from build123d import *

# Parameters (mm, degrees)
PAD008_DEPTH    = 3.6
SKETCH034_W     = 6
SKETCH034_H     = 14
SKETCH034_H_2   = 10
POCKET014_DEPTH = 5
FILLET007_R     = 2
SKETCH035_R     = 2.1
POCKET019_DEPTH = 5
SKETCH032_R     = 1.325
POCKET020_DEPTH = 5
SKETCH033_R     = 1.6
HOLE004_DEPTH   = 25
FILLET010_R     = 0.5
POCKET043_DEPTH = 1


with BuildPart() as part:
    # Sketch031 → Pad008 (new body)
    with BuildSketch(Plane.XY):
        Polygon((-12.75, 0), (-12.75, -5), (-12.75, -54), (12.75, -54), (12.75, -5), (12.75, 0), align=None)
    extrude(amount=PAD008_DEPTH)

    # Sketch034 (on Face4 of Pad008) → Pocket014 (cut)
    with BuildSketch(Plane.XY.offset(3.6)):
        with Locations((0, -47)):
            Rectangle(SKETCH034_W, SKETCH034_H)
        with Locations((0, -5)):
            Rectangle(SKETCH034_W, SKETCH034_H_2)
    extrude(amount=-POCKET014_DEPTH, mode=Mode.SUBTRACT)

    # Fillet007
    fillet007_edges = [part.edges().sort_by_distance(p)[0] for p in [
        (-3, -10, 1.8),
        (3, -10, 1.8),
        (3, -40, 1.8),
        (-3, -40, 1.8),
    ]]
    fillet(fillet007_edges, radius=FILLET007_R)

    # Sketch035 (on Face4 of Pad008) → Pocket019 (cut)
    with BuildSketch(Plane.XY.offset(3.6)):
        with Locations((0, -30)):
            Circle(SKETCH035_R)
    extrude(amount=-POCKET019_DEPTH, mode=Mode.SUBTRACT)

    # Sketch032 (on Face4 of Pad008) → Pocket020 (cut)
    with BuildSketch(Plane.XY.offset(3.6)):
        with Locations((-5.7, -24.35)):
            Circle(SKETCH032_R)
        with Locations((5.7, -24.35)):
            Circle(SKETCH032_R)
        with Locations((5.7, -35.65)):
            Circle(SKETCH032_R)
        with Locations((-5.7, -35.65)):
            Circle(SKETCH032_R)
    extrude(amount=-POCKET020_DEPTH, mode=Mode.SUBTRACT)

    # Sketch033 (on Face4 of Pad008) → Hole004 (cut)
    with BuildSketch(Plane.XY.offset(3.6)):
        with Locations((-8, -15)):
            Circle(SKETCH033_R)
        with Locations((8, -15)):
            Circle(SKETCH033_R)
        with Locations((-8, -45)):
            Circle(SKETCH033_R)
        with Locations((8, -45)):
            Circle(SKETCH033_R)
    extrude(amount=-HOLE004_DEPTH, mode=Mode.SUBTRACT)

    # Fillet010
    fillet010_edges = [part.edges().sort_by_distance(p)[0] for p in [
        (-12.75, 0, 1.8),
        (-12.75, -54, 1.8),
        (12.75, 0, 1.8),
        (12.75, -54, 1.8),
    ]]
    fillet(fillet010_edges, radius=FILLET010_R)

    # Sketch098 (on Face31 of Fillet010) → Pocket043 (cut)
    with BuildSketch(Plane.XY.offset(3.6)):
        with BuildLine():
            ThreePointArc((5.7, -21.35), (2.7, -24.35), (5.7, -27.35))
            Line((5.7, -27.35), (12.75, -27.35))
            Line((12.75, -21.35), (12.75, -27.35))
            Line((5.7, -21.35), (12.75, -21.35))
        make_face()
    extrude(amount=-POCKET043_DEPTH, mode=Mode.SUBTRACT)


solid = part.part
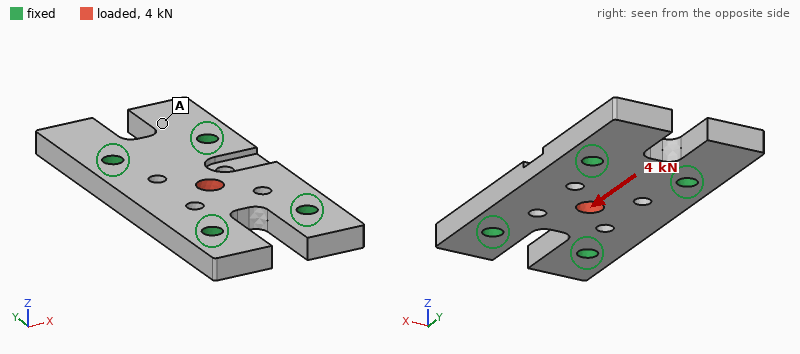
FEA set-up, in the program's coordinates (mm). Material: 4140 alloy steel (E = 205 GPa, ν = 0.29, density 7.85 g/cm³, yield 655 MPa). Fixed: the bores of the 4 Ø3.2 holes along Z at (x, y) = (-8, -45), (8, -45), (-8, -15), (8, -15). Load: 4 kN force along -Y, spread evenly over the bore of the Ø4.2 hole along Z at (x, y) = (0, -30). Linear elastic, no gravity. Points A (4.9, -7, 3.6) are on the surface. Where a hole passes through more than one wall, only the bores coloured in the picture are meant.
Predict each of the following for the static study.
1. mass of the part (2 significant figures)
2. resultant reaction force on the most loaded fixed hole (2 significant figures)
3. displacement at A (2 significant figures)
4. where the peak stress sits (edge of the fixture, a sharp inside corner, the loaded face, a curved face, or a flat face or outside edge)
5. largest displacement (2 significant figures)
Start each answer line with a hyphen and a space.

- 33 g
- 1.1 kN
- 0.64 µm
- the loaded face
- 4.0 µm
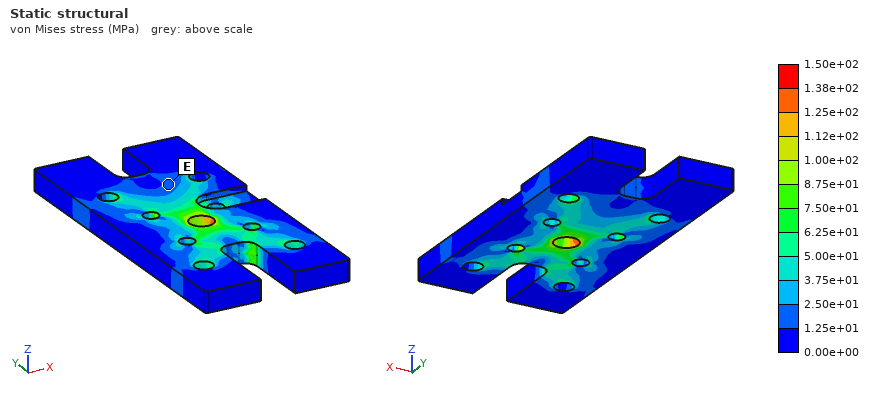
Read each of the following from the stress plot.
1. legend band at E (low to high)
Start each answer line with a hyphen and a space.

- 1.25e+01 to 2.50e+01 MPa
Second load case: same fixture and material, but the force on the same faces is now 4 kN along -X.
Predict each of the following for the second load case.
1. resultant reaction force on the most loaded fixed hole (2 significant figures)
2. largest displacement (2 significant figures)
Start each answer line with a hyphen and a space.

- 1.4 kN
- 7.3 µm
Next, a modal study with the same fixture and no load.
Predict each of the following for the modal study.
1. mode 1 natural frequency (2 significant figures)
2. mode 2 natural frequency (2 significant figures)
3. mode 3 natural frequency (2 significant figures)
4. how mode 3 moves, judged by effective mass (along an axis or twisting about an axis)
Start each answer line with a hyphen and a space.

- 14 kHz
- 15 kHz
- 20 kHz
- along Z
